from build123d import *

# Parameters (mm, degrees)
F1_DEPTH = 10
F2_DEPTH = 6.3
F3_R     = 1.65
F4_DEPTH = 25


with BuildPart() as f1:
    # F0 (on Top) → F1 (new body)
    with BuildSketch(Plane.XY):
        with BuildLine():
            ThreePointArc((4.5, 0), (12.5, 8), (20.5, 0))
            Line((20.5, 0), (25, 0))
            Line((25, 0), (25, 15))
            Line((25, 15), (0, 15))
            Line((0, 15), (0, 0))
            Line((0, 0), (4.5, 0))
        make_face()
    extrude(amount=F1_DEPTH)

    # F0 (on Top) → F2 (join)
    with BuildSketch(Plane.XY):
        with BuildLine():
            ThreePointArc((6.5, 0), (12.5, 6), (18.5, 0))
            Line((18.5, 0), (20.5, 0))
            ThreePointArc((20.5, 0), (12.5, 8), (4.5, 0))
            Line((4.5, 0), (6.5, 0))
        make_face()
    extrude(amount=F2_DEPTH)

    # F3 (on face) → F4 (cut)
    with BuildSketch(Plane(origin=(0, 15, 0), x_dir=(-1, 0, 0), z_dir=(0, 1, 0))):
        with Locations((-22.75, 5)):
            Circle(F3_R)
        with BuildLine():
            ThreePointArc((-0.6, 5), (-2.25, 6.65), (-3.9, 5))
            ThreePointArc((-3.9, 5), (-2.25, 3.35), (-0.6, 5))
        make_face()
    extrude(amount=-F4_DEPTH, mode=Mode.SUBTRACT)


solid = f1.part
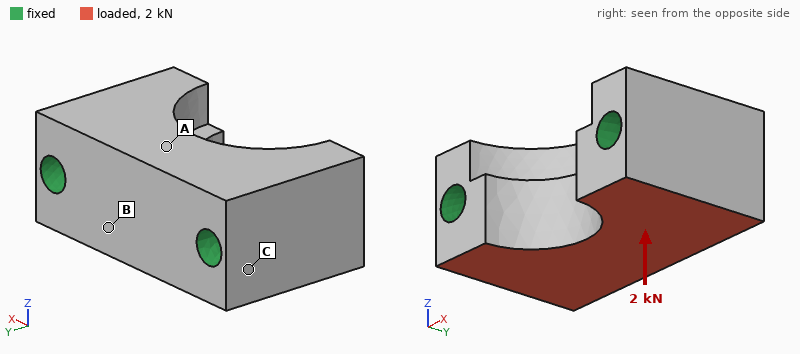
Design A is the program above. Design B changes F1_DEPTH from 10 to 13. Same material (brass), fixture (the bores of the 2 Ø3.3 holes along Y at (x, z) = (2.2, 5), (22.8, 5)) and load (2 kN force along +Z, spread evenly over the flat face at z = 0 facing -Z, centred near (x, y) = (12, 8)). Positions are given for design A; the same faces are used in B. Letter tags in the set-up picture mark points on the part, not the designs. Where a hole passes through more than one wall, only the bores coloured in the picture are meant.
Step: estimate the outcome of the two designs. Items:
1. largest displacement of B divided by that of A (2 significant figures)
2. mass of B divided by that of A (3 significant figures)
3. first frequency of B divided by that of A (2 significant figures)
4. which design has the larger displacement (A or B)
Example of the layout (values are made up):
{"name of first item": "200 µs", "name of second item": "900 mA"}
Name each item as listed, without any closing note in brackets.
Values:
{"largest displacement of B divided by that of A": "0.82", "mass of B divided by that of A": "1.30", "first frequency of B divided by that of A": "0.95", "which design has the larger displacement": "A"}
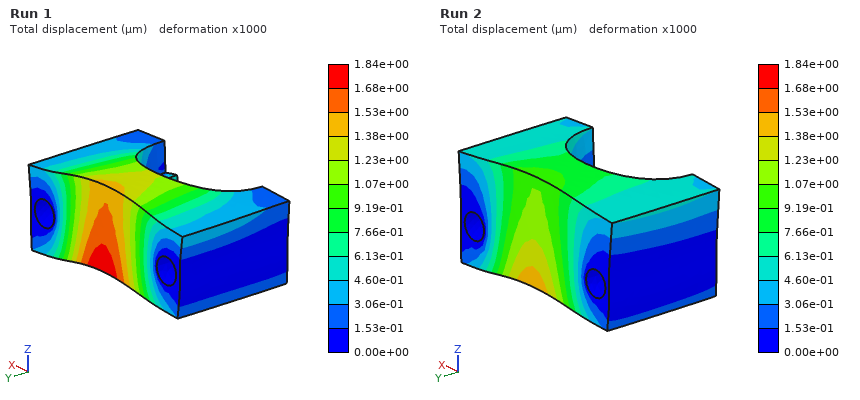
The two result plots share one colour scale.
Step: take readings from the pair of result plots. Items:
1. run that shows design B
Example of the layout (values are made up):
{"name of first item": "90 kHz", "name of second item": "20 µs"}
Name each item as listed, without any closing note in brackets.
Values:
{"run that shows design B": "Run 2"}
